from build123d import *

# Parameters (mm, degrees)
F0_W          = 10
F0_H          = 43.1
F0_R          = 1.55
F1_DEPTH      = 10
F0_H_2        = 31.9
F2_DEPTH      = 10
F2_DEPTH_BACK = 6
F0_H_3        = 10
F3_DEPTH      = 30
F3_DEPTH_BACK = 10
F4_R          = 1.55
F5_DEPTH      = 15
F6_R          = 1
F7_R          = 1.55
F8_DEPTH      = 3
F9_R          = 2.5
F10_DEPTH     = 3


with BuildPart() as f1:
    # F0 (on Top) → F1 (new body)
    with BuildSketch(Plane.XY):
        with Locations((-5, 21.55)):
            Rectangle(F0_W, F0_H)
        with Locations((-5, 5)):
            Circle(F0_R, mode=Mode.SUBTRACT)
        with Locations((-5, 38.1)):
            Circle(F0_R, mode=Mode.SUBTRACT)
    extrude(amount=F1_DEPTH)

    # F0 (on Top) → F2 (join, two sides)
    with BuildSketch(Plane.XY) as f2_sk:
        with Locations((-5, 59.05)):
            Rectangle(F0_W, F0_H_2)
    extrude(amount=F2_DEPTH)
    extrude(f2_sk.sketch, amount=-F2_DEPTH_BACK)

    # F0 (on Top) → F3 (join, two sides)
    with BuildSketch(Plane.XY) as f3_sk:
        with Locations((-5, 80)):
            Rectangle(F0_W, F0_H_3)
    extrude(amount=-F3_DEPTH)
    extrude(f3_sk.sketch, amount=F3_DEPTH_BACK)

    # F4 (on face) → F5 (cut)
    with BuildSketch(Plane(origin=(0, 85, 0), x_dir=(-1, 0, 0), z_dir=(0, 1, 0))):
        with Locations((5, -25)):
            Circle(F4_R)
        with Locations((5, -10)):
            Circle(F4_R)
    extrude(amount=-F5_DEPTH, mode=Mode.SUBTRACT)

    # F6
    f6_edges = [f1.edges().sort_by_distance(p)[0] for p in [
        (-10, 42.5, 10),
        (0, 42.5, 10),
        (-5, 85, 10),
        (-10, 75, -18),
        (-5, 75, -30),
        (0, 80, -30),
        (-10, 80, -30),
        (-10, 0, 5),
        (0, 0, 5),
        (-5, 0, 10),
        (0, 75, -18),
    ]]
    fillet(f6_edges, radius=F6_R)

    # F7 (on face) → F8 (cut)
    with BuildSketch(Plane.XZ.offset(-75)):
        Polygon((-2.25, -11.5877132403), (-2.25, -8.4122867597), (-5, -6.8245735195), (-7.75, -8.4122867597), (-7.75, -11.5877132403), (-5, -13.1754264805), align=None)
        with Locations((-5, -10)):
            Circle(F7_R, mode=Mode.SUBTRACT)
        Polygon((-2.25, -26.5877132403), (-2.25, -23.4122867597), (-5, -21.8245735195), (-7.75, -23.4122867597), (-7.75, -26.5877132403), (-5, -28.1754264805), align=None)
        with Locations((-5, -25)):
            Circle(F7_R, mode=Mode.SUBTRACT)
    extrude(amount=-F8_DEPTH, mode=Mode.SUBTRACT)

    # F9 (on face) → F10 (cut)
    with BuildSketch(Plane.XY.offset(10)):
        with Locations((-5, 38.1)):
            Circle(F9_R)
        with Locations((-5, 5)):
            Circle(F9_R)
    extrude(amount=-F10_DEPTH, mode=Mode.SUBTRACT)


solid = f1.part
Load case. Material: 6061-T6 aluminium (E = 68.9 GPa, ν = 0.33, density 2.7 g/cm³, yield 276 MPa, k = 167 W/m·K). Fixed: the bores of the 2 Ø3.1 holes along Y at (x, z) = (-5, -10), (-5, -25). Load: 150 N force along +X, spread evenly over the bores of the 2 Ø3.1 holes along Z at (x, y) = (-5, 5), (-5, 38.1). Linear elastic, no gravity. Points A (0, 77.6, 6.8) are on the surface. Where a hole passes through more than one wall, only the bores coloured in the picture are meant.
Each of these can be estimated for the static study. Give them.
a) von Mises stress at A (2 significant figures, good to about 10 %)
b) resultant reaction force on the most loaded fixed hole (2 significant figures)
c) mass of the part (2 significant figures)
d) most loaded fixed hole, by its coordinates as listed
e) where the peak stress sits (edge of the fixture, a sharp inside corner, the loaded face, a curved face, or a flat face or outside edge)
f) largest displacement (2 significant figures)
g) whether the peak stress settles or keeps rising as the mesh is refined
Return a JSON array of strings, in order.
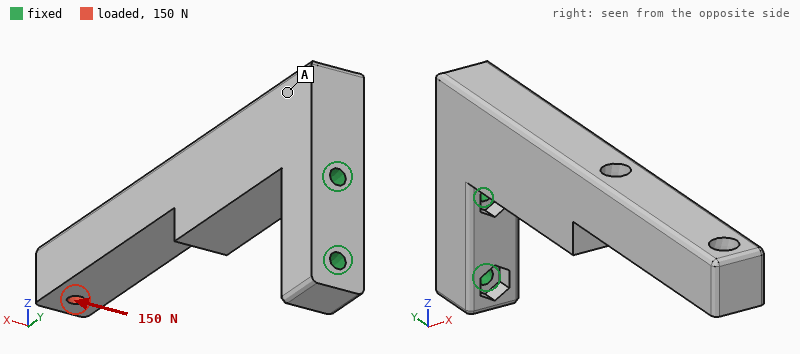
["15 MPa", "220 N", "35 g", "(-5, -10)", "edge of the fixture", "0.38 mm", "keeps rising"]
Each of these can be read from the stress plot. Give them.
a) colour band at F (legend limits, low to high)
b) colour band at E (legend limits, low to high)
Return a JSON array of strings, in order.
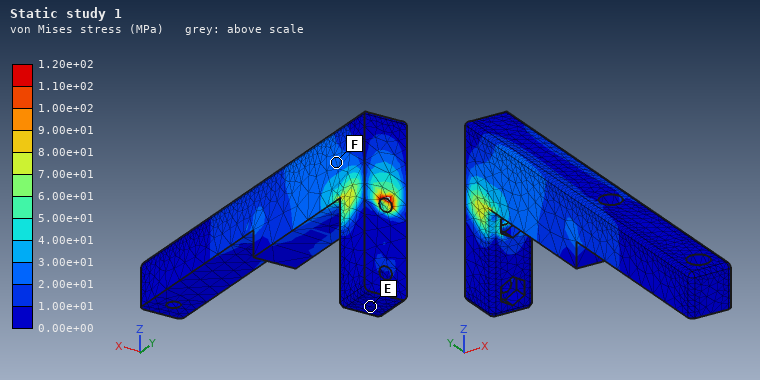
["2.00e+01 to 3.00e+01 MPa", "0.00e+00 to 1.00e+01 MPa"]
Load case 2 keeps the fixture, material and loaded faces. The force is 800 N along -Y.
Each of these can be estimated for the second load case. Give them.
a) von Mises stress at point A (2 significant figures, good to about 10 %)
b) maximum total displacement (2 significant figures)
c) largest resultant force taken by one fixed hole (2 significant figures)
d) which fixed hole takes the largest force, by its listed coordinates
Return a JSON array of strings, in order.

["6.7 MPa", "0.15 mm", "1.1 kN", "(-5, -10)"]
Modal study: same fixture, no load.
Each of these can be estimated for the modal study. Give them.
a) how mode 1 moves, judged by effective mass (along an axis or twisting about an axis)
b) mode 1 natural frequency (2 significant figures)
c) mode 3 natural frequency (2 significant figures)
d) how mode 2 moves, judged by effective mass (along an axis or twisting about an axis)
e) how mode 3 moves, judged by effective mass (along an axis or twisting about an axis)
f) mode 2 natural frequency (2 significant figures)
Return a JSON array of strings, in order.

["along X", "1100 Hz", "5400 Hz", "along Z", "along X", "1300 Hz"]
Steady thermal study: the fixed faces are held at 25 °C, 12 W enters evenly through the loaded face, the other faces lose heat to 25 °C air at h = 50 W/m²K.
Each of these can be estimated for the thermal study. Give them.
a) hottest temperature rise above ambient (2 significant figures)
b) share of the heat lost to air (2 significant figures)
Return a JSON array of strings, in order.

["32 K", "29 %"]
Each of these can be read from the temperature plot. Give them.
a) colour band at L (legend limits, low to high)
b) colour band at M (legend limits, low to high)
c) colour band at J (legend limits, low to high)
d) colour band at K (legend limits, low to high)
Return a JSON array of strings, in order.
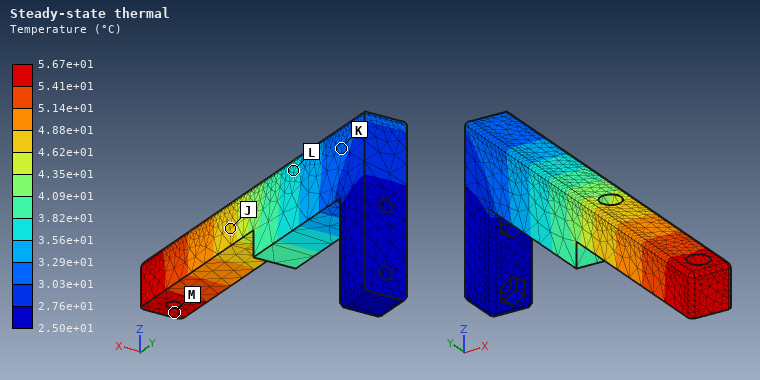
["3.56e+01 to 3.82e+01 °C", "5.41e+01 to 5.67e+01 °C", "4.62e+01 to 4.88e+01 °C", "3.03e+01 to 3.29e+01 °C"]
